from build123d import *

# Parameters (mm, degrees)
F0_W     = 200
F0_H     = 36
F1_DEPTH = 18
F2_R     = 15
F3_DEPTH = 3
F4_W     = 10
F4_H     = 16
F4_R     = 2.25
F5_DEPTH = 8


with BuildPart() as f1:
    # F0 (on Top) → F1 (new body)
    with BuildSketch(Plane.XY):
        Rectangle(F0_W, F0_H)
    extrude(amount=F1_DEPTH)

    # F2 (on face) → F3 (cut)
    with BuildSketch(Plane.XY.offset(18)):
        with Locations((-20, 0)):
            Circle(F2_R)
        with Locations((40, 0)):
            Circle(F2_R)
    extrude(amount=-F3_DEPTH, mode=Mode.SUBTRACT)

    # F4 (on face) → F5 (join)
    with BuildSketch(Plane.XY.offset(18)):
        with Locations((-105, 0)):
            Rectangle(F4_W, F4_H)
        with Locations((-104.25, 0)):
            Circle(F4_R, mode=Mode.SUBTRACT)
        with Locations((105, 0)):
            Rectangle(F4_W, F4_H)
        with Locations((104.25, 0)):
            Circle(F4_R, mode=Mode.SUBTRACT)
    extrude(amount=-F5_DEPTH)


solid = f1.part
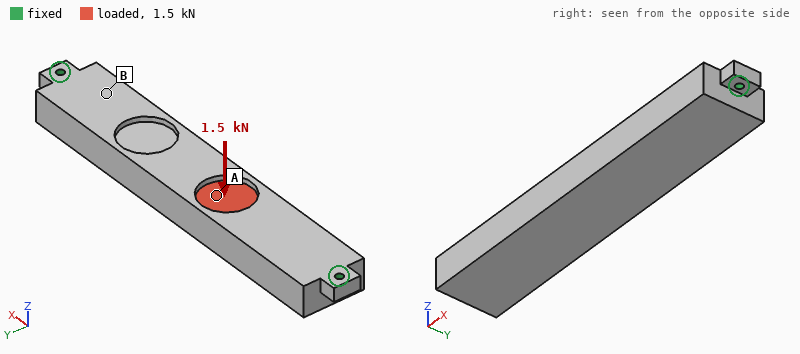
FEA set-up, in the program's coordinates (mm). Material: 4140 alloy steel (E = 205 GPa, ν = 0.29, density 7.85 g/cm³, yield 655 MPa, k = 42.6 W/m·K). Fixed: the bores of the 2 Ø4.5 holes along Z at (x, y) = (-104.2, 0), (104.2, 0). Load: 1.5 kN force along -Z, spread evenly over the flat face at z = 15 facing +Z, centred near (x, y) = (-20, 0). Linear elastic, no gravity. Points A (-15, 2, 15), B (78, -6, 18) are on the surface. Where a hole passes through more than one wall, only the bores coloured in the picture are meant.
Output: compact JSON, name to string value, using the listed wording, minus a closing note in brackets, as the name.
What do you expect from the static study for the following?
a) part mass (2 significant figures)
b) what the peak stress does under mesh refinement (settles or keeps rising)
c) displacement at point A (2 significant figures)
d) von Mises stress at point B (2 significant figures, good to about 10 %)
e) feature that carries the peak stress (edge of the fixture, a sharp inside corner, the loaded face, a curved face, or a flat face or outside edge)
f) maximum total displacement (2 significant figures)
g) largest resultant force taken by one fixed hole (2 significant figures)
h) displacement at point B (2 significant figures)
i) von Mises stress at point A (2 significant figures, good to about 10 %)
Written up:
{"part mass": "1.0 kg", "what the peak stress does under mesh refinement": "keeps rising", "displacement at point A": "46 µm", "von Mises stress at point B": "7.8 MPa", "feature that carries the peak stress": "edge of the fixture", "maximum total displacement": "46 µm", "largest resultant force taken by one fixed hole": "2.6 kN", "displacement at point B": "12 µm", "von Mises stress at point A": "21 MPa"}
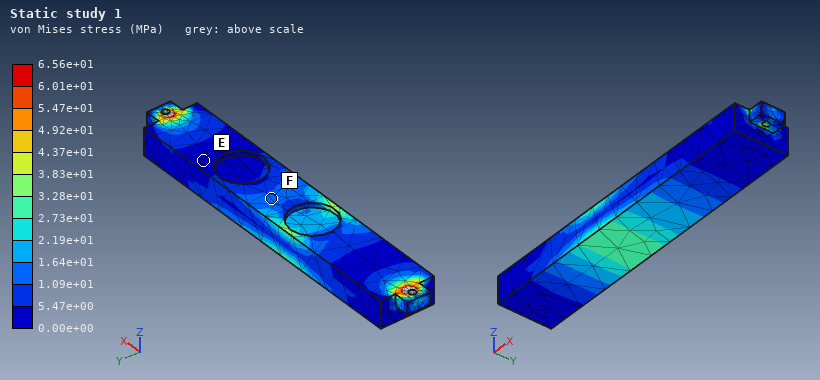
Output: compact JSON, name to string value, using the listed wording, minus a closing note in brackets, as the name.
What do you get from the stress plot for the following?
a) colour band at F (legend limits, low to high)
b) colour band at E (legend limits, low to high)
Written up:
{"colour band at F": "1.09e+01 to 1.64e+01 MPa", "colour band at E": "0.00e+00 to 5.47e+00 MPa"}
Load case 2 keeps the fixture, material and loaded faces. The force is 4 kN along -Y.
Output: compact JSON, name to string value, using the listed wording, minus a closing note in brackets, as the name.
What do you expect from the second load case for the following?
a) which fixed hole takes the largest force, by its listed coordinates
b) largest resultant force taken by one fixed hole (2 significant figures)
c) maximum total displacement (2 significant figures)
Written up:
{"which fixed hole takes the largest force, by its listed coordinates": "(-104.2, 0)", "largest resultant force taken by one fixed hole": "2.4 kN", "maximum total displacement": "52 µm"}
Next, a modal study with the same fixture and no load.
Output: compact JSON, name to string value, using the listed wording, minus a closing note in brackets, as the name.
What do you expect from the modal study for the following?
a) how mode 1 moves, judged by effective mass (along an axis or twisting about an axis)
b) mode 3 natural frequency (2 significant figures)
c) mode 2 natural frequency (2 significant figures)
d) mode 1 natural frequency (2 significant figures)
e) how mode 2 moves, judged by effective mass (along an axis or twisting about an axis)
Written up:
{"how mode 1 moves, judged by effective mass": "along Z", "mode 3 natural frequency": "2900 Hz", "mode 2 natural frequency": "1900 Hz", "mode 1 natural frequency": "1300 Hz", "how mode 2 moves, judged by effective mass": "along Y"}
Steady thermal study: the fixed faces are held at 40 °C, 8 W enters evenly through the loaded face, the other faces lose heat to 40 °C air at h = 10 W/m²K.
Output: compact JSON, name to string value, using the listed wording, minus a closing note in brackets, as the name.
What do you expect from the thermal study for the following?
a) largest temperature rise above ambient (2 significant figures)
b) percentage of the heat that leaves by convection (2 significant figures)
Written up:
{"largest temperature rise above ambient": "17 K", "percentage of the heat that leaves by convection": "26 %"}
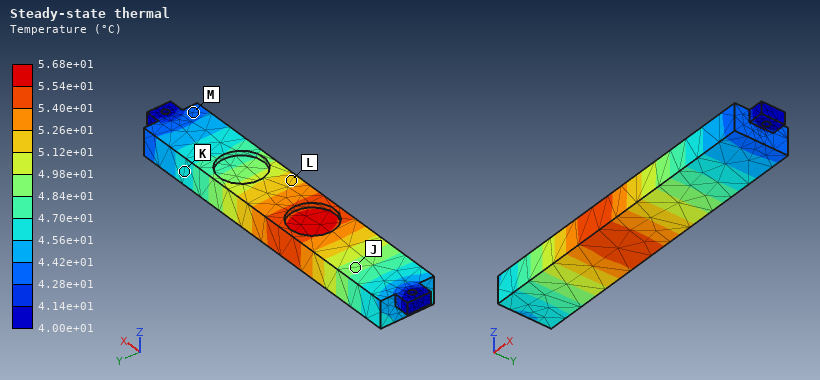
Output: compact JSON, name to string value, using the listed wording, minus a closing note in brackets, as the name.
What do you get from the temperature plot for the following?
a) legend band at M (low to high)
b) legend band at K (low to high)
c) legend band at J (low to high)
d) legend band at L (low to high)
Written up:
{"legend band at M": "4.28e+01 to 4.42e+01 °C", "legend band at K": "4.56e+01 to 4.70e+01 °C", "legend band at J": "4.84e+01 to 4.98e+01 °C", "legend band at L": "5.12e+01 to 5.26e+01 °C"}
